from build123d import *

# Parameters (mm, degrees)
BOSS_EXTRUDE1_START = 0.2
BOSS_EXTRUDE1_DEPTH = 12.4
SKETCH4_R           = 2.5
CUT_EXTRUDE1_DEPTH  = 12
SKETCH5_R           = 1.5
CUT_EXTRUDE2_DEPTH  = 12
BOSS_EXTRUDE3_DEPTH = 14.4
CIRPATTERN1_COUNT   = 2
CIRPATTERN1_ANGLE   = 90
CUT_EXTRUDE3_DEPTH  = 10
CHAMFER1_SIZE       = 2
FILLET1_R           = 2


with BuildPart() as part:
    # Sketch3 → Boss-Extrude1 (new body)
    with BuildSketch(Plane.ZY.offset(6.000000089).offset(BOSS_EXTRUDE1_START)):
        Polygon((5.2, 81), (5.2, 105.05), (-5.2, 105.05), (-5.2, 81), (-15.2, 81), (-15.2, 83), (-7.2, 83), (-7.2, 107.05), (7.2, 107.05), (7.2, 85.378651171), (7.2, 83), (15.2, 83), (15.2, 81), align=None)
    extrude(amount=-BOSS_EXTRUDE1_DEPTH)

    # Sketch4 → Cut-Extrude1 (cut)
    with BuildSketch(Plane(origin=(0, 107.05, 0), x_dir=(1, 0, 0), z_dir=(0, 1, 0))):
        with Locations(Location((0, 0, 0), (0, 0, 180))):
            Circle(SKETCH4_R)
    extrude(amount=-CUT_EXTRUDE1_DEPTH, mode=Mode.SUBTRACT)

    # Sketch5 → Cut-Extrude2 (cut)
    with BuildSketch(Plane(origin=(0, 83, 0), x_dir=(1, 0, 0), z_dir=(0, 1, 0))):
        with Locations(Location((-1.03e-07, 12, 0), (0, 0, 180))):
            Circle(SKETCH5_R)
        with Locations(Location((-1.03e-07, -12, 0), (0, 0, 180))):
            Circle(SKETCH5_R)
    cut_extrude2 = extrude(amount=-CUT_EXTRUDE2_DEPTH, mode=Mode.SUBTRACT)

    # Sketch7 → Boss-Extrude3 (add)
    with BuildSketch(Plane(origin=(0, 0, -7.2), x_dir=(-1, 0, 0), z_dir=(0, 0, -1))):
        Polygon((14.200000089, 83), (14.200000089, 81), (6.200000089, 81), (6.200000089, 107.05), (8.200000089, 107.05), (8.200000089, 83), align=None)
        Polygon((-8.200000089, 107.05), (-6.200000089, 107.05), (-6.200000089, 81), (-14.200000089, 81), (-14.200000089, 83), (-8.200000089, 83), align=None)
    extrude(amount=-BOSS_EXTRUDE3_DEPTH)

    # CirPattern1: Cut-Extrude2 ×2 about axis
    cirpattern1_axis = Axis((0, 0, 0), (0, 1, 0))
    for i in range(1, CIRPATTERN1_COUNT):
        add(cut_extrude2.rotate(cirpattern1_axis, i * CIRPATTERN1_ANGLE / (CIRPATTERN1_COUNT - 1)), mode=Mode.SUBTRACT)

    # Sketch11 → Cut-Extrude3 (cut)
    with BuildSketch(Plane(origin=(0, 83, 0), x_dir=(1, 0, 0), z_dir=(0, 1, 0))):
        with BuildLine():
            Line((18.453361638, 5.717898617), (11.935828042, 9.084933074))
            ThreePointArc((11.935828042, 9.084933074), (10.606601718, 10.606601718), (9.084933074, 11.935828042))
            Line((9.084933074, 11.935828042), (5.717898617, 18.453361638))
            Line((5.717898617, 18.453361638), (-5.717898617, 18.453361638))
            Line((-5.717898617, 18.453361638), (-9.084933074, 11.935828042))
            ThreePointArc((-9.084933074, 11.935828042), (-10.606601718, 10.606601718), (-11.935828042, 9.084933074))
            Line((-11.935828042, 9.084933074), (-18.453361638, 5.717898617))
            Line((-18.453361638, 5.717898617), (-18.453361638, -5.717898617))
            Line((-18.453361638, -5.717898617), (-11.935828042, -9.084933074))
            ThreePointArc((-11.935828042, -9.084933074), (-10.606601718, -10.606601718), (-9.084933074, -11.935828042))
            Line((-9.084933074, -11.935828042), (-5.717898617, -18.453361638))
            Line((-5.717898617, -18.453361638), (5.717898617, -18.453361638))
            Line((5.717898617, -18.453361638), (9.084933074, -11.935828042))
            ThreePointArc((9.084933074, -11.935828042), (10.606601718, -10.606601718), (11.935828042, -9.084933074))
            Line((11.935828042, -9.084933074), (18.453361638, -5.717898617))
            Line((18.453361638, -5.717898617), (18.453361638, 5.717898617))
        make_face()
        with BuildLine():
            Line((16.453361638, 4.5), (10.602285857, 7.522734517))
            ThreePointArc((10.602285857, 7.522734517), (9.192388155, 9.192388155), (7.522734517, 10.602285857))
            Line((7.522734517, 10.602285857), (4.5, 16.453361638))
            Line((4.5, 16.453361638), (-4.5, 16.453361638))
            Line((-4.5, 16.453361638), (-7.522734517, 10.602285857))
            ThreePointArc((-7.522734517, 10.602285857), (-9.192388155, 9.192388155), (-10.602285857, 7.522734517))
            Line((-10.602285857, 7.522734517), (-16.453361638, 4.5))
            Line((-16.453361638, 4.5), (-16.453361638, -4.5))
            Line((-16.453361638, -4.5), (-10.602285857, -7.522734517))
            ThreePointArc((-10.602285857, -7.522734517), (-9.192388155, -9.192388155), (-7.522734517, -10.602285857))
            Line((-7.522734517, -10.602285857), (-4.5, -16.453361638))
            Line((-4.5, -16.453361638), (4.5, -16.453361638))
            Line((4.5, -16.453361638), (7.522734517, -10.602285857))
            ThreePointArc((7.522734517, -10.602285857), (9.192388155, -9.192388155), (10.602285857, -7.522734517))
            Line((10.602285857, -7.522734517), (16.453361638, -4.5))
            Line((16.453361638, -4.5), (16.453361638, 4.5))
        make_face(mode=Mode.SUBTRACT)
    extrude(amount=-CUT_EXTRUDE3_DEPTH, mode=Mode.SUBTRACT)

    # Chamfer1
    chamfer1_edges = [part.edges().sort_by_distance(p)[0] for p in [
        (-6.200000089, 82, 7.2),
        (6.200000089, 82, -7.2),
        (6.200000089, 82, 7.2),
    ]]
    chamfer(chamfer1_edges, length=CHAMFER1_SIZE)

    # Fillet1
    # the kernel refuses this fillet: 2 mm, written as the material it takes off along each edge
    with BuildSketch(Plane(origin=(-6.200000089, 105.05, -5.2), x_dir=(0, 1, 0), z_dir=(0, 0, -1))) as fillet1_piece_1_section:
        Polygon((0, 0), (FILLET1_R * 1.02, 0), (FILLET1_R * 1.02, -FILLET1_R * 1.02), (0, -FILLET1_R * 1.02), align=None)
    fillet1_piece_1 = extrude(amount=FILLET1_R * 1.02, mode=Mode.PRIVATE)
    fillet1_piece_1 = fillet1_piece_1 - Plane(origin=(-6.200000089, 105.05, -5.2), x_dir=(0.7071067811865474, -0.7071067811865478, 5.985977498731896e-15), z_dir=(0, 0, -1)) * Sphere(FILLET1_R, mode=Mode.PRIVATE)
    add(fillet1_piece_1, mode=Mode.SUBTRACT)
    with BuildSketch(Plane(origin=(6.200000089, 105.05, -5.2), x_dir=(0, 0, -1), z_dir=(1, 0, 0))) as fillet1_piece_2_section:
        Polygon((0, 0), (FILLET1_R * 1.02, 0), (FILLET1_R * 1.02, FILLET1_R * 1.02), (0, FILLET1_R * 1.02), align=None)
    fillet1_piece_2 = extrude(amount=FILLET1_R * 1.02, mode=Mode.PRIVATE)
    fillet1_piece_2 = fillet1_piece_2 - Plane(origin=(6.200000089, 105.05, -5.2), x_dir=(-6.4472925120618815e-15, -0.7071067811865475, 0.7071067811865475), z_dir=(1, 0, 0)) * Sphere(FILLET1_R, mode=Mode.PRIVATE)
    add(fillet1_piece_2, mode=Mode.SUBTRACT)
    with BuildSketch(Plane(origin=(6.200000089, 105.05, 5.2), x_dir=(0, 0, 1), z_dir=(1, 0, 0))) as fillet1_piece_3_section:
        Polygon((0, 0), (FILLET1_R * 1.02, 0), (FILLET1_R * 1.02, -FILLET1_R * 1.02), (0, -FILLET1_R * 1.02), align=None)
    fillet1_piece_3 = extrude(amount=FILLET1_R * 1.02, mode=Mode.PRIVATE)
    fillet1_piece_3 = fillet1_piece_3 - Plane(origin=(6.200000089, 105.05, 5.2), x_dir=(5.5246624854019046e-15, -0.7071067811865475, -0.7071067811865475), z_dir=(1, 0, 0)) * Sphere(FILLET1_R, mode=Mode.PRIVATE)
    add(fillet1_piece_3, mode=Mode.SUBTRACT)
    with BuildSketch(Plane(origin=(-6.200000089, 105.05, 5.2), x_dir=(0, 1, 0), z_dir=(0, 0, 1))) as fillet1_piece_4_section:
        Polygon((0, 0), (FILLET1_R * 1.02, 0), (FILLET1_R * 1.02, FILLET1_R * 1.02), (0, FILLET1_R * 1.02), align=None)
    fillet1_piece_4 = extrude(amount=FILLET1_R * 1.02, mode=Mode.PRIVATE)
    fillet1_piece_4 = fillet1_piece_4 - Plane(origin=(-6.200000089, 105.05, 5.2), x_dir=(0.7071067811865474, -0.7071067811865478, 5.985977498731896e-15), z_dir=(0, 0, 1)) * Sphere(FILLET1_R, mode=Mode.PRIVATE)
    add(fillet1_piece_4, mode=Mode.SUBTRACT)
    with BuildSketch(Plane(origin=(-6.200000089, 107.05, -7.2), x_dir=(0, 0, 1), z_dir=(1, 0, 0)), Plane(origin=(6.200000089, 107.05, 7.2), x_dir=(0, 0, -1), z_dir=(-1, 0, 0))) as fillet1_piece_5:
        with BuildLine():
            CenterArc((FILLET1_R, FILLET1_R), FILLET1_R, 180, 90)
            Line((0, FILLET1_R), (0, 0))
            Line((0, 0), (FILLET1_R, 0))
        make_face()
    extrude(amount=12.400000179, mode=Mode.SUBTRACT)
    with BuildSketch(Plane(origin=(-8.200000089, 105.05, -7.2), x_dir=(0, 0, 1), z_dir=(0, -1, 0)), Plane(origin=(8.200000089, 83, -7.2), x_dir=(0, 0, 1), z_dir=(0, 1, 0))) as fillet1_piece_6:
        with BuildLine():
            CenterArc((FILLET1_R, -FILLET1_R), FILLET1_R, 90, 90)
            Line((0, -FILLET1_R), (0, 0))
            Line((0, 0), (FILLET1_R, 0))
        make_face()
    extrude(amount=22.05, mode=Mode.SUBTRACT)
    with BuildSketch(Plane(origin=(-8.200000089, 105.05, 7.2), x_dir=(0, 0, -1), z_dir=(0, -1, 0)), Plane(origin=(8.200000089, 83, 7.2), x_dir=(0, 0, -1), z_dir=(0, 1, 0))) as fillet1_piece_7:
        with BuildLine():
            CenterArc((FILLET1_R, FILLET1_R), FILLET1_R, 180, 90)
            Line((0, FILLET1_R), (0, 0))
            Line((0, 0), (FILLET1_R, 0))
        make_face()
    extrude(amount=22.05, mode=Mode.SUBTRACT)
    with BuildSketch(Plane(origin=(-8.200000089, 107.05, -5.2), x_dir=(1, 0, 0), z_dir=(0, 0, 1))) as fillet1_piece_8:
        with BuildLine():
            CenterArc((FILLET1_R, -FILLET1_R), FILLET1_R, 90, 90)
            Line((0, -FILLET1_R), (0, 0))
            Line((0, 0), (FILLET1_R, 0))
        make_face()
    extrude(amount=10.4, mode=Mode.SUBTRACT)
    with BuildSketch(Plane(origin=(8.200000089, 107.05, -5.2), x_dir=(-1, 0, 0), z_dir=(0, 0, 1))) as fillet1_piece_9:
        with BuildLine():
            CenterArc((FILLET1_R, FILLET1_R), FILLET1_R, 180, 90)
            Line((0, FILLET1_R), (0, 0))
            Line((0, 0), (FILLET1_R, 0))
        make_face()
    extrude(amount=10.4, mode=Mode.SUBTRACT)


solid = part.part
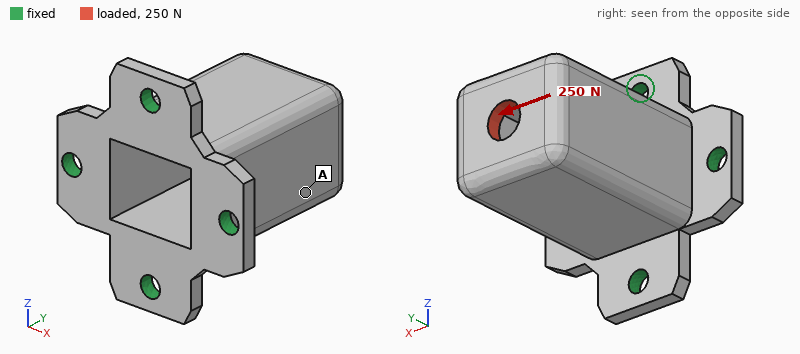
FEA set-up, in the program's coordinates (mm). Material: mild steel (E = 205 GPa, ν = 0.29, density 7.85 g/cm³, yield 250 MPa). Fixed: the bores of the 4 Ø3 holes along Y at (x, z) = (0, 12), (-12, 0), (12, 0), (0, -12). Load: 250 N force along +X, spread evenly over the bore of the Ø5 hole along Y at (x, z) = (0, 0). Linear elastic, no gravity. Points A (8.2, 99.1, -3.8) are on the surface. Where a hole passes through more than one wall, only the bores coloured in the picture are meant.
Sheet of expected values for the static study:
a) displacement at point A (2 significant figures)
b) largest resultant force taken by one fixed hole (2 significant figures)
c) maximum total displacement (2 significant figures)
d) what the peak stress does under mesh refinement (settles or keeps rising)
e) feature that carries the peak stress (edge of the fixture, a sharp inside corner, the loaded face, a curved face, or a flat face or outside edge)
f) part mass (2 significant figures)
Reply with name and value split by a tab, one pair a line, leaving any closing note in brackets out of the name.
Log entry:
displacement at point A	7.2 µm
largest resultant force taken by one fixed hole	310 N
maximum total displacement	10 µm
what the peak stress does under mesh refinement	keeps rising
feature that carries the peak stress	edge of the fixture
part mass	28 g
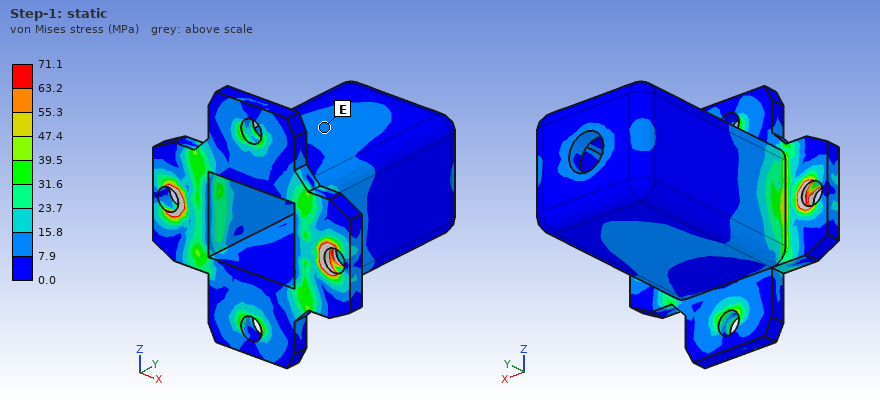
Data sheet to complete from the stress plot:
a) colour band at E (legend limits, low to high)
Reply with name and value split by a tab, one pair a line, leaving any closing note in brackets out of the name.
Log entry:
colour band at E	7.9 to 15.8 MPa
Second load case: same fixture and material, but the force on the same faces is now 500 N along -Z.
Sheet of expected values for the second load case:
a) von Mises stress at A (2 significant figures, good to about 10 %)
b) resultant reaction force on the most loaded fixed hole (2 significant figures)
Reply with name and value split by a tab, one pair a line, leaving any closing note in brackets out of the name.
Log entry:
von Mises stress at A	17 MPa
resultant reaction force on the most loaded fixed hole	610 N
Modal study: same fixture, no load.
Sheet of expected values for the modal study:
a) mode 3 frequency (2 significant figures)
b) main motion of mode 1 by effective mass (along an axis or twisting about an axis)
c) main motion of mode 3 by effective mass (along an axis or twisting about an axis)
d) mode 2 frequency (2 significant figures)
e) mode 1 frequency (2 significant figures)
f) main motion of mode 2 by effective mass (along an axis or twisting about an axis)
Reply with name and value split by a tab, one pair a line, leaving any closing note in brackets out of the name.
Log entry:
mode 3 frequency	19 kHz
main motion of mode 1 by effective mass	along Z
main motion of mode 3 by effective mass	along Y
mode 2 frequency	8400 Hz
mode 1 frequency	7000 Hz
main motion of mode 2 by effective mass	along X
